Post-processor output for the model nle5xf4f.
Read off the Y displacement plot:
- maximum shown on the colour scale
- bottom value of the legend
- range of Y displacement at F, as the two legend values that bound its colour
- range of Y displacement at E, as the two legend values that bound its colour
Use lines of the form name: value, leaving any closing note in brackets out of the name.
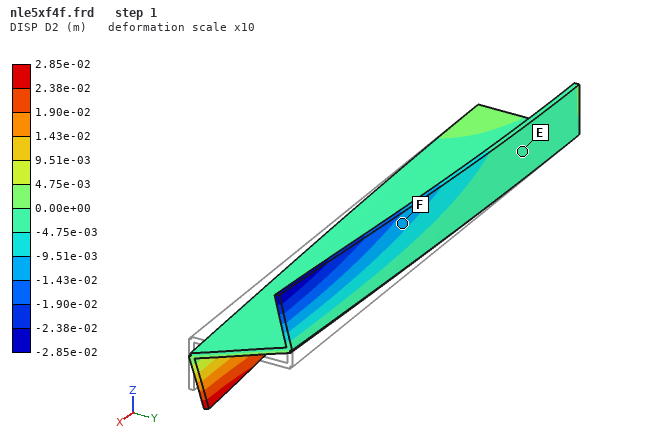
maximum shown on the colour scale: 2.85e-02 m
bottom value of the legend: -2.85e-02 m
range of Y displacement at F, as the two legend values that bound its colour: -1.43e-02 to -9.51e-03 m
range of Y displacement at E, as the two legend values that bound its colour: -4.75e-03 to 0.00e+00 m
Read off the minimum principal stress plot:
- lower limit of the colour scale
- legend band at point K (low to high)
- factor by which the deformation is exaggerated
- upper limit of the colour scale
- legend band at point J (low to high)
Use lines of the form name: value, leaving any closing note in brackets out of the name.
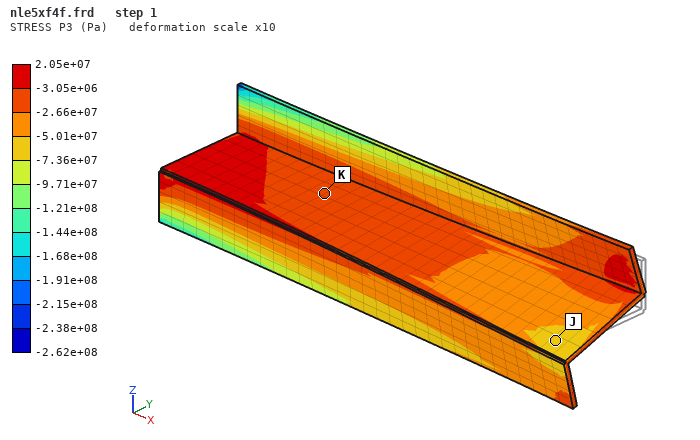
lower limit of the colour scale: -2.62e+08 Pa
legend band at point K: -2.66e+07 to -3.05e+06 Pa
factor by which the deformation is exaggerated: 10
upper limit of the colour scale: 2.05e+07 Pa
legend band at point J: -7.36e+07 to -5.01e+07 Pa
